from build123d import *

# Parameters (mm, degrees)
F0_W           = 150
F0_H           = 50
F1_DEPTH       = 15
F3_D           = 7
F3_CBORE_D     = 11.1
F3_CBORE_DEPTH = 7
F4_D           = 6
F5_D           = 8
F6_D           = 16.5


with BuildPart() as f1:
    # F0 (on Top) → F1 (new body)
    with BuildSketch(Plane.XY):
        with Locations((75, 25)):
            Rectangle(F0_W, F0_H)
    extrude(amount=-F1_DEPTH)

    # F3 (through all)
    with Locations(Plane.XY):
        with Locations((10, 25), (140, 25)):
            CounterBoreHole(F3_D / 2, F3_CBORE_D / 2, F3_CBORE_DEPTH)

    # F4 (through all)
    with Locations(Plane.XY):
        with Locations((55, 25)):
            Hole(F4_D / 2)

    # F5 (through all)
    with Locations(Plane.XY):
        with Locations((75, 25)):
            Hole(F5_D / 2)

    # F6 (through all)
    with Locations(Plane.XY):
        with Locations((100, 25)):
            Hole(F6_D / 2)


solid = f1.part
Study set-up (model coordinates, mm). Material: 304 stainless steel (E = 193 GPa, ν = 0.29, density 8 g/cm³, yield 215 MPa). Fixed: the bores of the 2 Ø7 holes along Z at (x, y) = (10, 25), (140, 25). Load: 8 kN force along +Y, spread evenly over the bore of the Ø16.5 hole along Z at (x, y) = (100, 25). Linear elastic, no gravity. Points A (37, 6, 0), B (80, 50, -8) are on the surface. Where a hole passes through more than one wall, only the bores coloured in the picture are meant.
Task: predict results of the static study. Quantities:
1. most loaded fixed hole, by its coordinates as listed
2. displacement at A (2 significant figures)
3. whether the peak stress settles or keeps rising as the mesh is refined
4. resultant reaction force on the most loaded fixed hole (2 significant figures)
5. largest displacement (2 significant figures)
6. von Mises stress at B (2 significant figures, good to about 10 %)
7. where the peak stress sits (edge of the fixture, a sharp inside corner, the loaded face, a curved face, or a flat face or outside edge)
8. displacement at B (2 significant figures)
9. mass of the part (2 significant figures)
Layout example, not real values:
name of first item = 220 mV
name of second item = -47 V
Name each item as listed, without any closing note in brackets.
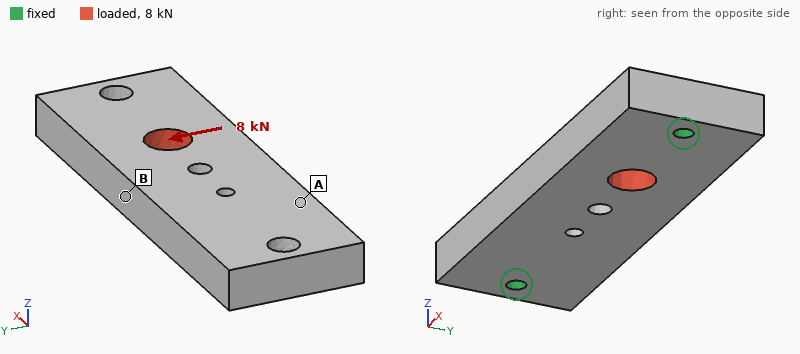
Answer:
most loaded fixed hole, by its coordinates as listed = (140, 25)
displacement at A = 9.1 µm
whether the peak stress settles or keeps rising as the mesh is refined = keeps rising
resultant reaction force on the most loaded fixed hole = 5.6 kN
largest displacement = 16 µm
von Mises stress at B = 28 MPa
where the peak stress sits = edge of the fixture
displacement at B = 14 µm
mass of the part = 850 g
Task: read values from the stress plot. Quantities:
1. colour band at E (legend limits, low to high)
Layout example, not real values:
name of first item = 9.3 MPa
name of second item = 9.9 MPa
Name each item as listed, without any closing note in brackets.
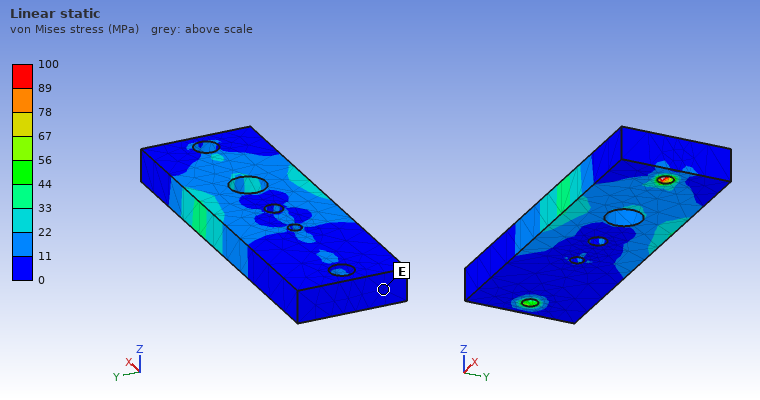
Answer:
colour band at E = 0 to 11 MPa
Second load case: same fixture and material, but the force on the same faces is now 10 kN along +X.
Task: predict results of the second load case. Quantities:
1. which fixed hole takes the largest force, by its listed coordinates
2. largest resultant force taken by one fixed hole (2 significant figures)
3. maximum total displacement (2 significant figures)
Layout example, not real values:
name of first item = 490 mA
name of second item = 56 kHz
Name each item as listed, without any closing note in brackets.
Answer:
which fixed hole takes the largest force, by its listed coordinates = (140, 25)
largest resultant force taken by one fixed hole = 6.1 kN
maximum total displacement = 5.1 µm
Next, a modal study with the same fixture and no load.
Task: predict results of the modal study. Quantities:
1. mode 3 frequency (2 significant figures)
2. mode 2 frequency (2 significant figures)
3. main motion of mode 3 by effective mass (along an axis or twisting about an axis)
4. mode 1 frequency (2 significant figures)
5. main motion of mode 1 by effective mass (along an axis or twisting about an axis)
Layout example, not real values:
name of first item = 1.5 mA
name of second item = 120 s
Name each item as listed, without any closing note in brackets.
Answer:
mode 3 frequency = 5800 Hz
mode 2 frequency = 3700 Hz
main motion of mode 3 by effective mass = along Y
mode 1 frequency = 2900 Hz
main motion of mode 1 by effective mass = along Z
